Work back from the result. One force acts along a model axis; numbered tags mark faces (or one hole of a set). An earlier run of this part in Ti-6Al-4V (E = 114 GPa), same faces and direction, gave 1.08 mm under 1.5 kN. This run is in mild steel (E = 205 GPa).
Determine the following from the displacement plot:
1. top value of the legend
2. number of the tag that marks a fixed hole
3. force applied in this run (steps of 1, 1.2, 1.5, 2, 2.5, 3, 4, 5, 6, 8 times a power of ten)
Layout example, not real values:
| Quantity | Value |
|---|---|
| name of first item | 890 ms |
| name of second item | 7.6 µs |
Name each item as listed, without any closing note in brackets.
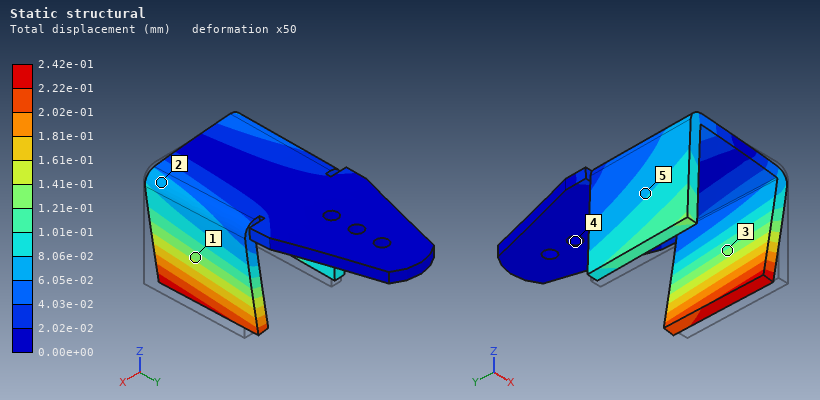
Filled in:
| Quantity | Value |
|---|---|
| top value of the legend | 2.42e-01 mm |
| number of the tag that marks a fixed hole | 4 |
| force applied in this run | 600 N |
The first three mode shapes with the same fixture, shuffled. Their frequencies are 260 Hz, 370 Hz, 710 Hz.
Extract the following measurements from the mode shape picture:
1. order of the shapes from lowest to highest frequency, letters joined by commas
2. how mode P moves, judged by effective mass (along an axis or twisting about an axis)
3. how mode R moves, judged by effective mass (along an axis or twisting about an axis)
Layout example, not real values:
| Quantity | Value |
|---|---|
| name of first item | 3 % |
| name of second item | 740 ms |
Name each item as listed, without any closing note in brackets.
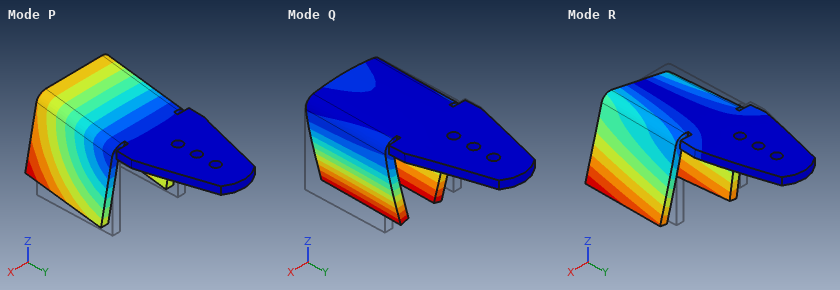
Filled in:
| Quantity | Value |
|---|---|
| order of the shapes from lowest to highest frequency, letters joined by commas | P, R, Q |
| how mode P moves, judged by effective mass | along Z |
| how mode R moves, judged by effective mass | along X |
